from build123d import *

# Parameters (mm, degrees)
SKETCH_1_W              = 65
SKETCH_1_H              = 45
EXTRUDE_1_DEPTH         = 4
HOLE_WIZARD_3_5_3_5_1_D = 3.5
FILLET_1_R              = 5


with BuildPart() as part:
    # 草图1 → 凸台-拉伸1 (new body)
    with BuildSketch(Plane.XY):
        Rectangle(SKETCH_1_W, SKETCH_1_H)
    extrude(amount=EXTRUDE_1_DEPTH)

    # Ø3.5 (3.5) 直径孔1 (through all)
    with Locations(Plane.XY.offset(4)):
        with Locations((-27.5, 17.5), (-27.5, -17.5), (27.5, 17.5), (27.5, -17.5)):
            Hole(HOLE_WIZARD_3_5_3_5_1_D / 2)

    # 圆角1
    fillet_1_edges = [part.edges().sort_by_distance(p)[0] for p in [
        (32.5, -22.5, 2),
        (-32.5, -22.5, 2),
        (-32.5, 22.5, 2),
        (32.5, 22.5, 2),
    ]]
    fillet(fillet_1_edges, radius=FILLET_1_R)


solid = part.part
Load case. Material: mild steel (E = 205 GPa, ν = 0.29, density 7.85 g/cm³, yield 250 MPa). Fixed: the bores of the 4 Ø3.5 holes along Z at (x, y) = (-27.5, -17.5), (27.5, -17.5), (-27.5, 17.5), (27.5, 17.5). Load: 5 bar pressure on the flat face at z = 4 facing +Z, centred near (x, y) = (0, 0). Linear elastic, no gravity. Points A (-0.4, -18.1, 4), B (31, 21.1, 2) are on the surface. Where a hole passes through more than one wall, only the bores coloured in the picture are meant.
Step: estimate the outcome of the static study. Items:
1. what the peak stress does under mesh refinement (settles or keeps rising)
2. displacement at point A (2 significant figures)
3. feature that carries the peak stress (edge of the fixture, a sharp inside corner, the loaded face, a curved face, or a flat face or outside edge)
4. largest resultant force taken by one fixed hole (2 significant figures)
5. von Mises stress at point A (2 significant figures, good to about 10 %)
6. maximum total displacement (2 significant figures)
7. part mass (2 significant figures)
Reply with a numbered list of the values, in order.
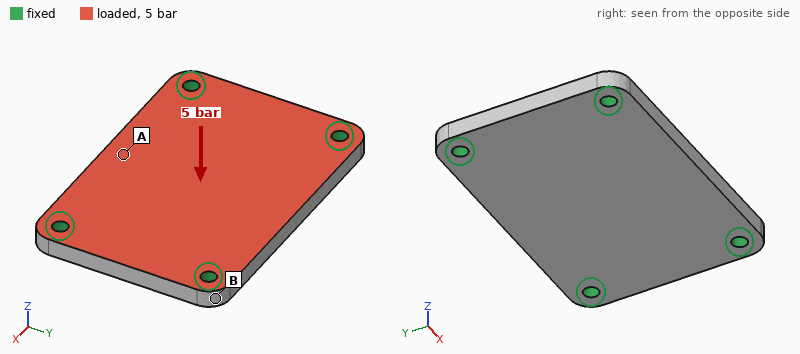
1. keeps rising
2. 14 µm
3. edge of the fixture
4. 360 N
5. 27 MPa
6. 16 µm
7. 90 g
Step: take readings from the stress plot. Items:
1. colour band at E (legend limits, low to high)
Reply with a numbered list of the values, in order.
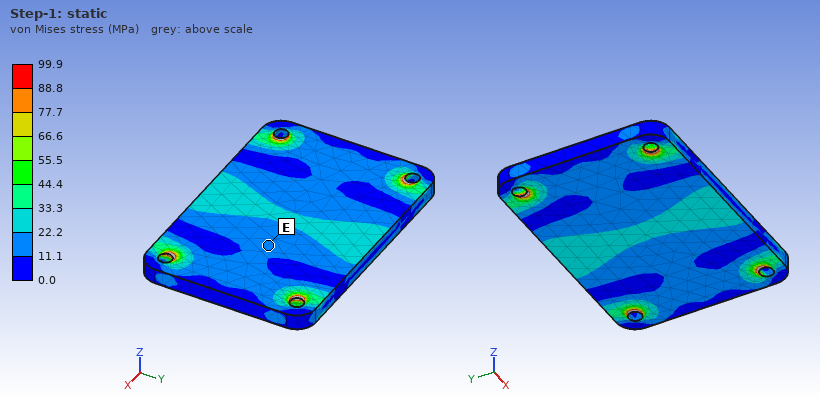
1. 11.1 to 22.2 MPa
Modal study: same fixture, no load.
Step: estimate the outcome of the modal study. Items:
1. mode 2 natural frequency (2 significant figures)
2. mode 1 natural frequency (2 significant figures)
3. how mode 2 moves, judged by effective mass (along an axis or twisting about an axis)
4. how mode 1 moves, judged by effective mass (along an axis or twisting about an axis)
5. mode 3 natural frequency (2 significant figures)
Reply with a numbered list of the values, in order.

1. 8700 Hz
2. 5900 Hz
3. twisting about X
4. along Z
5. 14 kHz
